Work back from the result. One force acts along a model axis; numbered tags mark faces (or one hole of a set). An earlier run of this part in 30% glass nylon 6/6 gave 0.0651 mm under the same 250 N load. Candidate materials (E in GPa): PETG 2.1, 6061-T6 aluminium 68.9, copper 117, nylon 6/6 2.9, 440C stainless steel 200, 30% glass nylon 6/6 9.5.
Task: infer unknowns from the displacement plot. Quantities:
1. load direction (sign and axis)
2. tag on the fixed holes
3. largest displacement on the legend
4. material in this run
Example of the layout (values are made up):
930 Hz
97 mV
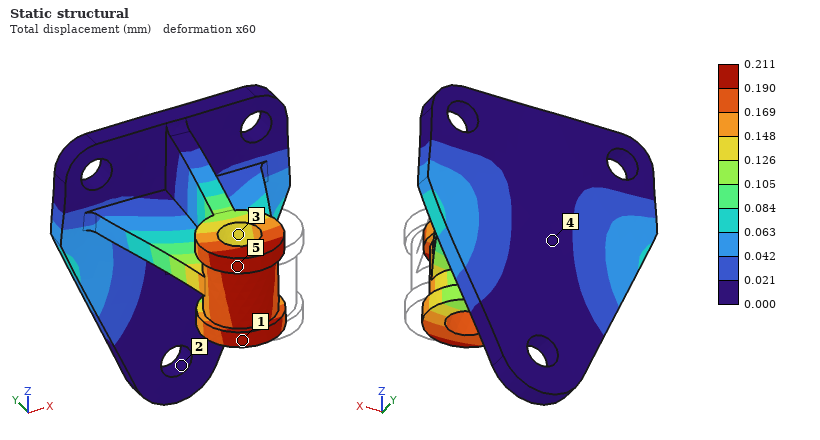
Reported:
-X
2
0.211 mm
nylon 6/6
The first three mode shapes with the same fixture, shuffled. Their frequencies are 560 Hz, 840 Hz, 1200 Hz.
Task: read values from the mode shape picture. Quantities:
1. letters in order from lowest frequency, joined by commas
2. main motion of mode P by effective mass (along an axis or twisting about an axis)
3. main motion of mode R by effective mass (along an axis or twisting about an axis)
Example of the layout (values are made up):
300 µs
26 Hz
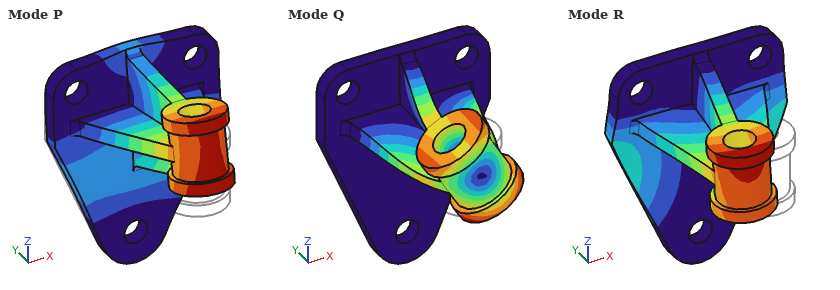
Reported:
P, R, Q
along Z
along X
